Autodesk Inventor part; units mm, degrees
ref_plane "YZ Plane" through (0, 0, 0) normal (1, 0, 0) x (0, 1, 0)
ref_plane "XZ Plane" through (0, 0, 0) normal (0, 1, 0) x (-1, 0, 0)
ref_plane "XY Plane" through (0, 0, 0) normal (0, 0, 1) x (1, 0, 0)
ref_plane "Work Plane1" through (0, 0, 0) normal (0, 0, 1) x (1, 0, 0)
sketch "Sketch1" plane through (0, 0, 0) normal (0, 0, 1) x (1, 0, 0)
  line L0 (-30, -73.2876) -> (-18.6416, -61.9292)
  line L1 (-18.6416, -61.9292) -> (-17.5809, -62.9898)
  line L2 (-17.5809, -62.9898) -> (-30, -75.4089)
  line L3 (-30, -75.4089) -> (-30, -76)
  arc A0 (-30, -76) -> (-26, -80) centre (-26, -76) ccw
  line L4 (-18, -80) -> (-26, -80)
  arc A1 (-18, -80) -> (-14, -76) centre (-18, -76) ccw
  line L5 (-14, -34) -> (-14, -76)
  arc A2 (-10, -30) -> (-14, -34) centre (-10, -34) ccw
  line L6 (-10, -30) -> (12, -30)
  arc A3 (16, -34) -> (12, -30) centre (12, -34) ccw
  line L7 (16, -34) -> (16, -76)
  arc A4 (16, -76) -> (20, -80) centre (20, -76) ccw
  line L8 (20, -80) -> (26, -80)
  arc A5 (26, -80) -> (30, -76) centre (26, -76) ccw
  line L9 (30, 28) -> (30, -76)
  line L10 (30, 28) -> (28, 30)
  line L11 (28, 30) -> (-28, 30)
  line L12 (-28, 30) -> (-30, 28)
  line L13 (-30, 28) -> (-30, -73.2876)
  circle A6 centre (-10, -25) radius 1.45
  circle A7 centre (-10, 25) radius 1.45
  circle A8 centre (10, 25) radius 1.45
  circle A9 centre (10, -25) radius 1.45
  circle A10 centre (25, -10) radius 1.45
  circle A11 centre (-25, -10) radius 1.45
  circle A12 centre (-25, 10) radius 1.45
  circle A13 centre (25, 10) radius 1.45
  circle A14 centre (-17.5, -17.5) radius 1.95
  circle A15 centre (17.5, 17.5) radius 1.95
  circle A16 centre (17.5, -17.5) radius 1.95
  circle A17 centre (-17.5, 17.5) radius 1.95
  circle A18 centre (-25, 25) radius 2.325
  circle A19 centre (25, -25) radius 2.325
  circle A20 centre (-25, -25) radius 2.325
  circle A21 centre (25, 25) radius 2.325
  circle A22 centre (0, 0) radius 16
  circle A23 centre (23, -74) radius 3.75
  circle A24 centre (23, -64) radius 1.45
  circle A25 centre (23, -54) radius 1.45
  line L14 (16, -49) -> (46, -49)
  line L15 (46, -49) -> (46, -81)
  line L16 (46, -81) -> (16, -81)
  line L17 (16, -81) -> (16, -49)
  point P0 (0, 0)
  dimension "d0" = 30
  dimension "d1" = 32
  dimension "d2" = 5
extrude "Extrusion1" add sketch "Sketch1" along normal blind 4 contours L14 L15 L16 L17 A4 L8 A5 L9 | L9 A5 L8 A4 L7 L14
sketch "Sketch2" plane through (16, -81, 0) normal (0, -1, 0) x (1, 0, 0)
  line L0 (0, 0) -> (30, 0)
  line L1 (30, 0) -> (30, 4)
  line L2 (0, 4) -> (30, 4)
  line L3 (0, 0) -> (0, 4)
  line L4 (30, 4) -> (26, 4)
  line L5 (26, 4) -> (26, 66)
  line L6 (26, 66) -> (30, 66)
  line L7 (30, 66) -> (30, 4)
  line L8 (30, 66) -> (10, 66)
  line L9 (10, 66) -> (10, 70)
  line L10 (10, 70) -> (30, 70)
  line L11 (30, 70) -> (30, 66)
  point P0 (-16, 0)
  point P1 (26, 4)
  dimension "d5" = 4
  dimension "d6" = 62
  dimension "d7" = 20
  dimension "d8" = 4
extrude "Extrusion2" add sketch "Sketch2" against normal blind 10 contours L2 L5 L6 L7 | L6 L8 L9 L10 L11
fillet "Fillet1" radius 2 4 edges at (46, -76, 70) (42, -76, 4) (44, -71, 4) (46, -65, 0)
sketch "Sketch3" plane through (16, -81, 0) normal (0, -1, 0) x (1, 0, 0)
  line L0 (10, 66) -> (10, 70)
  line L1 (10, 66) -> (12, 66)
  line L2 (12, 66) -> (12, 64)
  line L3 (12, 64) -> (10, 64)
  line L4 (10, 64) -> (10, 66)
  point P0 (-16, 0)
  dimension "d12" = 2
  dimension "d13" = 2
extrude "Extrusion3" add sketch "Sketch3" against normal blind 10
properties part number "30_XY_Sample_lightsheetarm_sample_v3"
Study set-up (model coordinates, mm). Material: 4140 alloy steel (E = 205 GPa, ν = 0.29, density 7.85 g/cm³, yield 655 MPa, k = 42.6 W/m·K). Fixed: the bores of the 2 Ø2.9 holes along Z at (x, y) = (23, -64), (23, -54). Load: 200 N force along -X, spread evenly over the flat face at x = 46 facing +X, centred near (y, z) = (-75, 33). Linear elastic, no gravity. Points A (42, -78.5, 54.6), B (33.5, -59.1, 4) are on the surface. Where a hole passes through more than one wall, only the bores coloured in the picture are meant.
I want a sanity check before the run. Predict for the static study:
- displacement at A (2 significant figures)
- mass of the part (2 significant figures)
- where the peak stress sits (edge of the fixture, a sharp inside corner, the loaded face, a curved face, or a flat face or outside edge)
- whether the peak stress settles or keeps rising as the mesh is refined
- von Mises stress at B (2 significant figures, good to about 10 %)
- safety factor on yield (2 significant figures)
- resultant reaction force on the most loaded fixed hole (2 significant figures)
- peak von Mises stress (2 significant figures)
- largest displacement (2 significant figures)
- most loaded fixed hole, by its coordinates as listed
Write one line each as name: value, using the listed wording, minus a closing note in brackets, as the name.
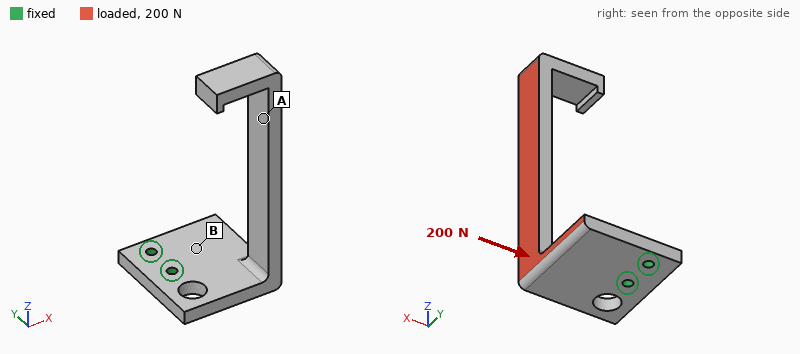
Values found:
displacement at A: 0.70 mm
mass of the part: 54 g
where the peak stress sits: a curved face
whether the peak stress settles or keeps rising as the mesh is refined: settles
von Mises stress at B: 68 MPa
safety factor on yield: 1.7
resultant reaction force on the most loaded fixed hole: 370 N
peak von Mises stress: 380 MPa
largest displacement: 0.99 mm
most loaded fixed hole, by its coordinates as listed: (23, -64)
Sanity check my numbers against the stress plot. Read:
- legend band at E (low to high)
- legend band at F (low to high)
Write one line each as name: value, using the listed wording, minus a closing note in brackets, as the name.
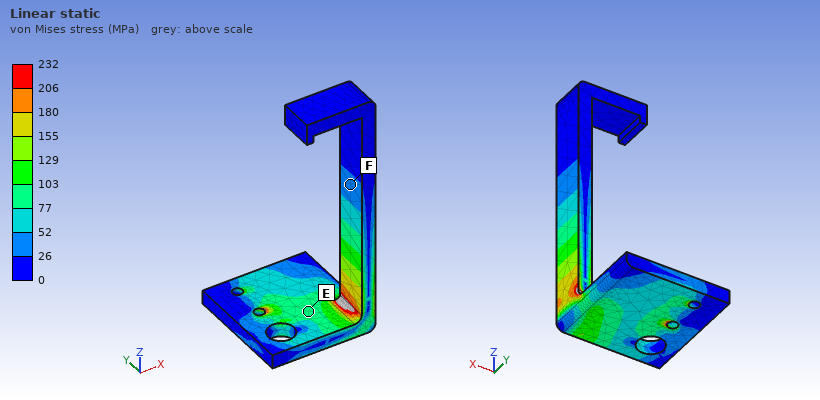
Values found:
legend band at E: 77 to 103 MPa
legend band at F: 26 to 52 MPa
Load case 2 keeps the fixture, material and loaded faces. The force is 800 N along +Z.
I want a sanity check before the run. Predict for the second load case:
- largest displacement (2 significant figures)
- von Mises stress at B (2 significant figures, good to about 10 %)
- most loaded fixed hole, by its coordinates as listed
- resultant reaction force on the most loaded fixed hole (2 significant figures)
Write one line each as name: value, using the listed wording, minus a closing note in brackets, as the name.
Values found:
largest displacement: 0.94 mm
von Mises stress at B: 170 MPa
most loaded fixed hole, by its coordinates as listed: (23, -64)
resultant reaction force on the most loaded fixed hole: 1.2 kN
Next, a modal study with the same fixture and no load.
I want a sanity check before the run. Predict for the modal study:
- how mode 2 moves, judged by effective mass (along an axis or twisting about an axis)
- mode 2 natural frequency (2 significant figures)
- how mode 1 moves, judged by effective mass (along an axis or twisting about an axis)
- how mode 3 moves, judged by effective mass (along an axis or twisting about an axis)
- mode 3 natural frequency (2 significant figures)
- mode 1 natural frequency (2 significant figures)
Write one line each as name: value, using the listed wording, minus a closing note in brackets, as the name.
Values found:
how mode 2 moves, judged by effective mass: along Y
mode 2 natural frequency: 660 Hz
how mode 1 moves, judged by effective mass: along X
how mode 3 moves, judged by effective mass: along Z
mode 3 natural frequency: 2000 Hz
mode 1 natural frequency: 420 Hz
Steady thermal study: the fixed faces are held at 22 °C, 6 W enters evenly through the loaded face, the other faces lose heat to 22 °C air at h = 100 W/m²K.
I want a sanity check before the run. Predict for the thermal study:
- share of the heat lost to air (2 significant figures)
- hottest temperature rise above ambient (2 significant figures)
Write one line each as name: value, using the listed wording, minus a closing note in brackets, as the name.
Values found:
share of the heat lost to air: 77 %
hottest temperature rise above ambient: 29 K
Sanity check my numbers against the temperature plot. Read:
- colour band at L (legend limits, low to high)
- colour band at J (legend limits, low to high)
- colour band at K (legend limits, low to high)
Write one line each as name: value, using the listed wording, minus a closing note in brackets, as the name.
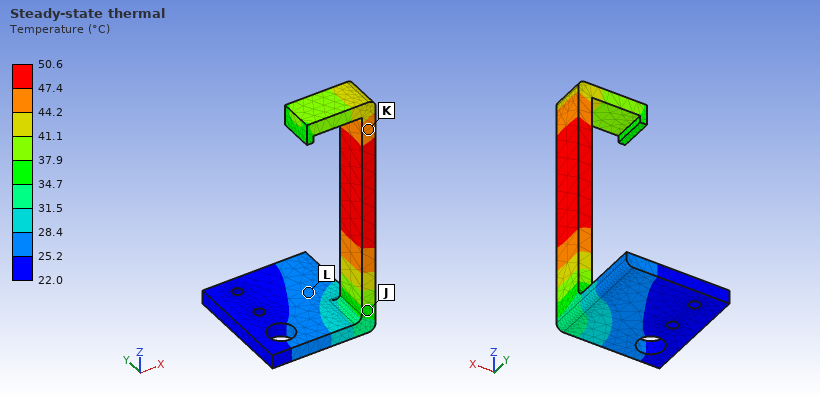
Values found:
colour band at L: 25.2 to 28.4 °C
colour band at J: 34.7 to 37.9 °C
colour band at K: 44.2 to 47.4 °C
